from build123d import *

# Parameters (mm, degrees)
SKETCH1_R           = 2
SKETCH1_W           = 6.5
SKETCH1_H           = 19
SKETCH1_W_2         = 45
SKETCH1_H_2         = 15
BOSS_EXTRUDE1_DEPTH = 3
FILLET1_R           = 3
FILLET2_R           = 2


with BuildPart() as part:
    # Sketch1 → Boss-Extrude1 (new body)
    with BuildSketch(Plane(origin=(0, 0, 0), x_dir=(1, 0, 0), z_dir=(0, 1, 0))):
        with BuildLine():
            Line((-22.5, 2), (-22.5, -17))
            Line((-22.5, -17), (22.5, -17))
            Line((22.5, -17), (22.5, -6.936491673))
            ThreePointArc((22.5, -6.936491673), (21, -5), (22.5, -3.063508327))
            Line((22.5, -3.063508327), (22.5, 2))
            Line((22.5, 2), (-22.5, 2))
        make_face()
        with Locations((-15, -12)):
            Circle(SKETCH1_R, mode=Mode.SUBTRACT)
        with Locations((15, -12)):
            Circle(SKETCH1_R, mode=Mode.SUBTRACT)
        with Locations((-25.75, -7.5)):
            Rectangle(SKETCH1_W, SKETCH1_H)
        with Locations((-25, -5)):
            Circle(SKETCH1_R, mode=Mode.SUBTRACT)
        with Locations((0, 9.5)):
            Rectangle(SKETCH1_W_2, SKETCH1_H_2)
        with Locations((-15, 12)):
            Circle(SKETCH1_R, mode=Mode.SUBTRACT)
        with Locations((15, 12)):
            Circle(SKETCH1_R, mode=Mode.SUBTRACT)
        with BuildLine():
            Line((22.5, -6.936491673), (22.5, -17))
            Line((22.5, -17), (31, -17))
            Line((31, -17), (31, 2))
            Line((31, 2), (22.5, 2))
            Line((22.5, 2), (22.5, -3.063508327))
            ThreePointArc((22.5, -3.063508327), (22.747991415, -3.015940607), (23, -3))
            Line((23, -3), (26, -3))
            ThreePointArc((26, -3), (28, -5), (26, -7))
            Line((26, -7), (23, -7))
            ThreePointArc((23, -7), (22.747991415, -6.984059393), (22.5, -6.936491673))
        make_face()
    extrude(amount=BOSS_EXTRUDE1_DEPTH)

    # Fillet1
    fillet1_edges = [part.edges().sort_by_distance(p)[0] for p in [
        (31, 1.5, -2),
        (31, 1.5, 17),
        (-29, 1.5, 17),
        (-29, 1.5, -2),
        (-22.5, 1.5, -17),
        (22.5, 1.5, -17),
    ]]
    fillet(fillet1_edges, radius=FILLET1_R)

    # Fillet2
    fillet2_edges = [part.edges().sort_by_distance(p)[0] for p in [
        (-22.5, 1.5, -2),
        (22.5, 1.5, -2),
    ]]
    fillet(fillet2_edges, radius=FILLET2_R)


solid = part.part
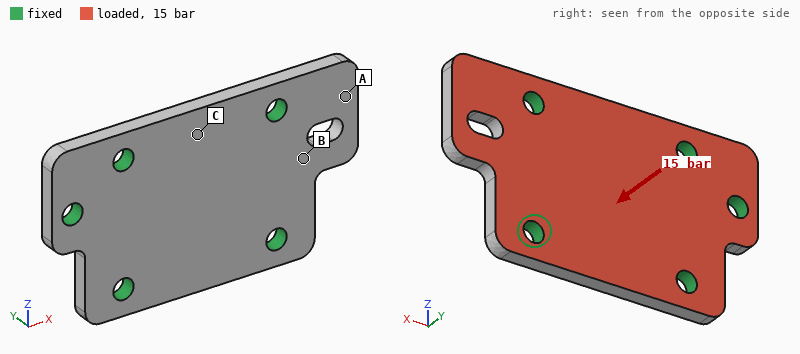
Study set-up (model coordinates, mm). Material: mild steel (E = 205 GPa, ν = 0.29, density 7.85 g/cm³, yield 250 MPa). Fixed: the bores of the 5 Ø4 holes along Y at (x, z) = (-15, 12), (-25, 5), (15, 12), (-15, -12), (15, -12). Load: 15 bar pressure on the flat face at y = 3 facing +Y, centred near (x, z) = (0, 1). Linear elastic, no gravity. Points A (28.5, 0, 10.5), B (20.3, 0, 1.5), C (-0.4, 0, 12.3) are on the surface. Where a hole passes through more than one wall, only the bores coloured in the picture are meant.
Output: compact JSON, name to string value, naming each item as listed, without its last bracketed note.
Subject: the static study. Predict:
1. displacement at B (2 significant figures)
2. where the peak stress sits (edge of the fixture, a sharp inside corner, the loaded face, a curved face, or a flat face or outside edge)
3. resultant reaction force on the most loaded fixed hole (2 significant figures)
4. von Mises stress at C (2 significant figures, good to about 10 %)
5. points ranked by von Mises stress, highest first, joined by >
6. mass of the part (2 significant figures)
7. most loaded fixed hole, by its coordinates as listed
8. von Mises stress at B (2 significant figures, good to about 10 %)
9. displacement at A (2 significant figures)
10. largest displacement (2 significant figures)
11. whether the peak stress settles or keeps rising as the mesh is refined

{"displacement at B": "6.4 µm", "where the peak stress sits": "edge of the fixture", "resultant reaction force on the most loaded fixed hole": "730 N", "von Mises stress at C": "34 MPa", "points ranked by von Mises stress, highest first, joined by >": "B > C > A", "mass of the part": "40 g", "most loaded fixed hole, by its coordinates as listed": "(15, 12)", "von Mises stress at B": "56 MPa", "displacement at A": "16 µm", "largest displacement": "21 µm", "whether the peak stress settles or keeps rising as the mesh is refined": "keeps rising"}
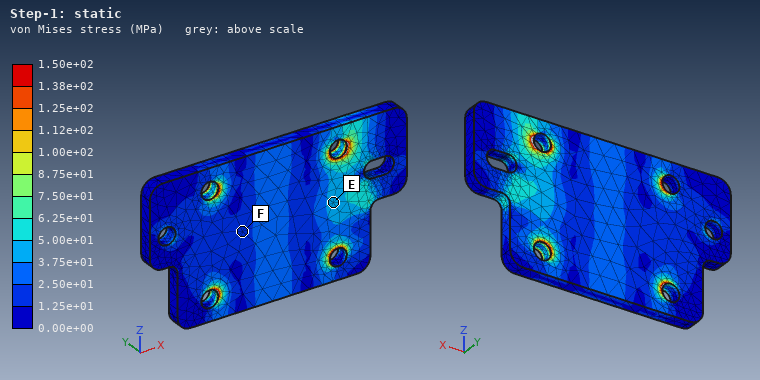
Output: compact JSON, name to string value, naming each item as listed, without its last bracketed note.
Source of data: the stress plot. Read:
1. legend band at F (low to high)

{"legend band at F": "1.25e+01 to 2.50e+01 MPa"}
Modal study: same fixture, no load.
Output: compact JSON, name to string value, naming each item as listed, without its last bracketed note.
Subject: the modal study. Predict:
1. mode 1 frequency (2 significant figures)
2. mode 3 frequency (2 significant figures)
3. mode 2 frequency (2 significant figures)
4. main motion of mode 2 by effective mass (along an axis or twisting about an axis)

{"mode 1 frequency": "11 kHz", "mode 3 frequency": "20 kHz", "mode 2 frequency": "16 kHz", "main motion of mode 2 by effective mass": "along Y"}
